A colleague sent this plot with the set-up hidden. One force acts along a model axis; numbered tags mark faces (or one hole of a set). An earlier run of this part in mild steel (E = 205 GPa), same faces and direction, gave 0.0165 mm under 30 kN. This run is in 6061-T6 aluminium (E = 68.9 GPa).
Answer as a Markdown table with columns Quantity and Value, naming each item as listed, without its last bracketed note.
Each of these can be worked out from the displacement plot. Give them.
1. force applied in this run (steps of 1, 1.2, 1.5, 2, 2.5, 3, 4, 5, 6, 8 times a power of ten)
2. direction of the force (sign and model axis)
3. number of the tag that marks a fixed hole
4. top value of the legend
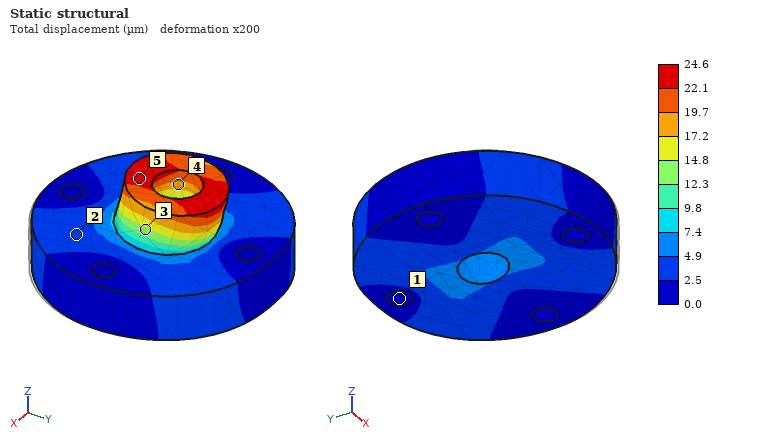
| Quantity | Value |
|---|---|
| force applied in this run | 15 kN |
| direction of the force | +Y |
| number of the tag that marks a fixed hole | 1 |
| top value of the legend | 24.6 µm |
